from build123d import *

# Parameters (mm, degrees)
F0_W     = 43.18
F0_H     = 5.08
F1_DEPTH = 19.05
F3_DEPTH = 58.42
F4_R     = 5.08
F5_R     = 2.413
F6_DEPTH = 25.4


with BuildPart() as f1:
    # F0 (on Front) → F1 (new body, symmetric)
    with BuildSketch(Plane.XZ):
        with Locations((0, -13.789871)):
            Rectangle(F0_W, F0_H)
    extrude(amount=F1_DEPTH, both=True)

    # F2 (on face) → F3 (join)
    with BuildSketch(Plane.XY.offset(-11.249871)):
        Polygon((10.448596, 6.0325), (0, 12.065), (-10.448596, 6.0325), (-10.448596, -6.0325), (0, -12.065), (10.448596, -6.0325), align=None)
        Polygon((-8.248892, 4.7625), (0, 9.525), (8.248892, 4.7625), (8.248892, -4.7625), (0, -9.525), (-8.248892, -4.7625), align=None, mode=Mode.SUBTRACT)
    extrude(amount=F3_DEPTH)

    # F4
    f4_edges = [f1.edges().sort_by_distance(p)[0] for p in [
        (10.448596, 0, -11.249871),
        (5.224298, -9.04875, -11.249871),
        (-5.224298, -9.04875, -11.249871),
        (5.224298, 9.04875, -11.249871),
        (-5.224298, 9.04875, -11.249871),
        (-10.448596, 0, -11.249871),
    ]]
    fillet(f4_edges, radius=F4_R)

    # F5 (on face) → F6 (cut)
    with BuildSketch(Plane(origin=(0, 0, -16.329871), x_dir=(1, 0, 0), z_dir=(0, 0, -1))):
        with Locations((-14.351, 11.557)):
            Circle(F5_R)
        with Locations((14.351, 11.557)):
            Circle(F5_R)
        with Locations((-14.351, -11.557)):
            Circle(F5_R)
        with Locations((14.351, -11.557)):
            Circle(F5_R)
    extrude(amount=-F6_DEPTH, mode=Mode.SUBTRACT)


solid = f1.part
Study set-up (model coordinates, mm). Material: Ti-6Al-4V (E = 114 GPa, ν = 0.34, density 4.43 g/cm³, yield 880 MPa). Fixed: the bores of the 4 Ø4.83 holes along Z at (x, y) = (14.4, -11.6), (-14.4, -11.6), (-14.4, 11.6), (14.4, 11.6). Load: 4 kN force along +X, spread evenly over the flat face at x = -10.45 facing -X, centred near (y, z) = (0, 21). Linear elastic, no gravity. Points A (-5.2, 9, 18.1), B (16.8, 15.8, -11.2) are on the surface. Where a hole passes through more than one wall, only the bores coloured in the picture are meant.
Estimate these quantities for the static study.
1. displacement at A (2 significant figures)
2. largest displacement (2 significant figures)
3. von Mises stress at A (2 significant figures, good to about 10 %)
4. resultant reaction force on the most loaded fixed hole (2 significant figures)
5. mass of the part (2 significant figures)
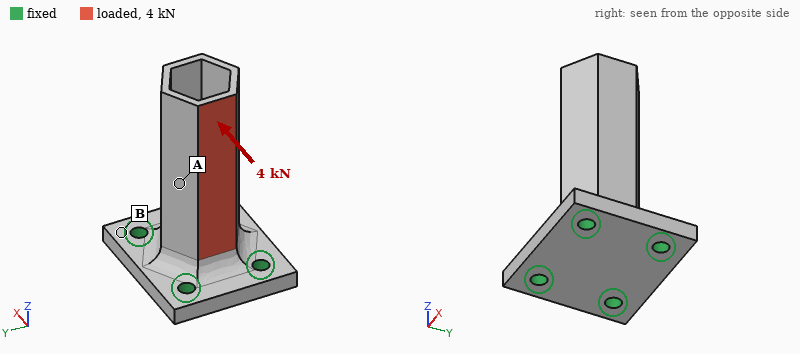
0.097 mm
0.24 mm
55 MPa
3.0 kN
74 g
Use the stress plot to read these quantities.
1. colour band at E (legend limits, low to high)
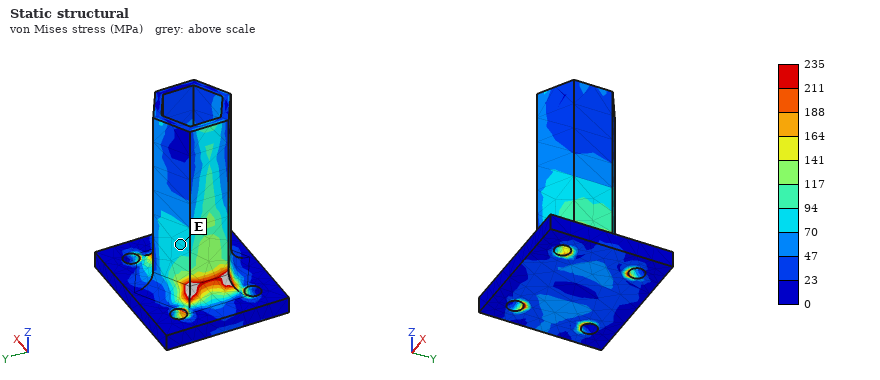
70 to 94 MPa
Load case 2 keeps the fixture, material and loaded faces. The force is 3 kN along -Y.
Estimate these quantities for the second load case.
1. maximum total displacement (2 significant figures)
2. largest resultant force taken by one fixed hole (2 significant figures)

0.20 mm
2.6 kN
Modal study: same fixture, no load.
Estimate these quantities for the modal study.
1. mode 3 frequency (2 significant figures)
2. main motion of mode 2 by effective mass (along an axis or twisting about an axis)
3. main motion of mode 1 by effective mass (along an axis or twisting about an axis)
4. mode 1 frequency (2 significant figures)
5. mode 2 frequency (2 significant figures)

13 kHz
along X
along Y
4200 Hz
4500 Hz
